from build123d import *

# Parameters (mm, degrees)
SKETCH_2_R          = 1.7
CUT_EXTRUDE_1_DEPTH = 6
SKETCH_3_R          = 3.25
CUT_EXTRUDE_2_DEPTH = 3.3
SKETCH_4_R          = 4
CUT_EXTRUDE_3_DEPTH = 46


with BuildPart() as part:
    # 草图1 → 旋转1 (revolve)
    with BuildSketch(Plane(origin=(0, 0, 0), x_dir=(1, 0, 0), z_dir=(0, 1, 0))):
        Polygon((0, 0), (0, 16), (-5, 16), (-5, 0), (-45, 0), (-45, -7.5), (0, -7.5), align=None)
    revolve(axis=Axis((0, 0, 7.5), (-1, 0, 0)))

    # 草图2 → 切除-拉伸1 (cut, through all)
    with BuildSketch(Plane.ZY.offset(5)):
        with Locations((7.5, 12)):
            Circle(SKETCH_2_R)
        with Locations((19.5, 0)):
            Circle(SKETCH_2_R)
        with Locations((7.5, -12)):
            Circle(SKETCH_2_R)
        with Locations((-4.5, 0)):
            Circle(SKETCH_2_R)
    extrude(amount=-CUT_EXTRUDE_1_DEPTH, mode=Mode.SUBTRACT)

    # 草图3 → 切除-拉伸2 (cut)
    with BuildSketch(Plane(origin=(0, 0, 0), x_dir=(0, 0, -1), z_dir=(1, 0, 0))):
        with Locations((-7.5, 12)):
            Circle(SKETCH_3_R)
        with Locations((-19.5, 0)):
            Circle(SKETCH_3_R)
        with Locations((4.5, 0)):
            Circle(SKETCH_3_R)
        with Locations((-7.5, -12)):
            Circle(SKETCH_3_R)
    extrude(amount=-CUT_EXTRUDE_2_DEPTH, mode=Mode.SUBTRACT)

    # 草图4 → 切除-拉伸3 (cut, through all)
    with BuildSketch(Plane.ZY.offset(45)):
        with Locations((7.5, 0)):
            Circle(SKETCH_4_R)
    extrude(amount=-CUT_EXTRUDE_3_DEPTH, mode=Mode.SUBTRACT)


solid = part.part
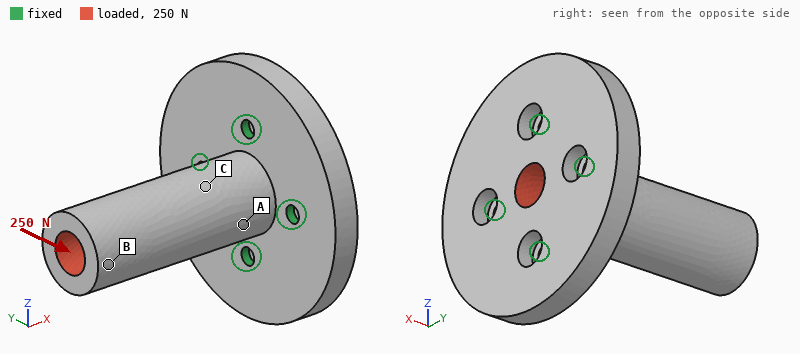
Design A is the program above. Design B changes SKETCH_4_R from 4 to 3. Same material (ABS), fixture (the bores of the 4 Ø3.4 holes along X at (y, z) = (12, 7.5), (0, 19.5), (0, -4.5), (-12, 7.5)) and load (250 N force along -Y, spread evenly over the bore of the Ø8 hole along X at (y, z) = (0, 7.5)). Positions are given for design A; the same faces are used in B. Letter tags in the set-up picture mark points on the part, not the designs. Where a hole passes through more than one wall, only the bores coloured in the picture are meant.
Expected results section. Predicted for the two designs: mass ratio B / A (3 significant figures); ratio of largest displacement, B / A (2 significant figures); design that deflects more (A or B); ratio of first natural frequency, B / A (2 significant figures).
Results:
1.08
0.91
A
0.97
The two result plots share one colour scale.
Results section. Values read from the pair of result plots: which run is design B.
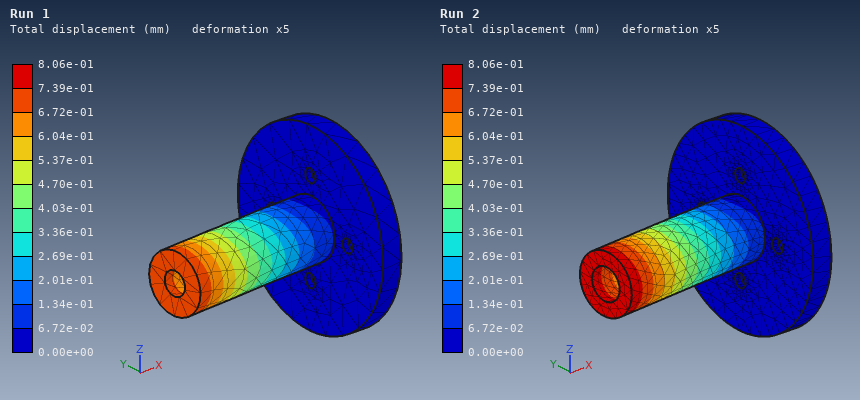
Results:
Run 1
